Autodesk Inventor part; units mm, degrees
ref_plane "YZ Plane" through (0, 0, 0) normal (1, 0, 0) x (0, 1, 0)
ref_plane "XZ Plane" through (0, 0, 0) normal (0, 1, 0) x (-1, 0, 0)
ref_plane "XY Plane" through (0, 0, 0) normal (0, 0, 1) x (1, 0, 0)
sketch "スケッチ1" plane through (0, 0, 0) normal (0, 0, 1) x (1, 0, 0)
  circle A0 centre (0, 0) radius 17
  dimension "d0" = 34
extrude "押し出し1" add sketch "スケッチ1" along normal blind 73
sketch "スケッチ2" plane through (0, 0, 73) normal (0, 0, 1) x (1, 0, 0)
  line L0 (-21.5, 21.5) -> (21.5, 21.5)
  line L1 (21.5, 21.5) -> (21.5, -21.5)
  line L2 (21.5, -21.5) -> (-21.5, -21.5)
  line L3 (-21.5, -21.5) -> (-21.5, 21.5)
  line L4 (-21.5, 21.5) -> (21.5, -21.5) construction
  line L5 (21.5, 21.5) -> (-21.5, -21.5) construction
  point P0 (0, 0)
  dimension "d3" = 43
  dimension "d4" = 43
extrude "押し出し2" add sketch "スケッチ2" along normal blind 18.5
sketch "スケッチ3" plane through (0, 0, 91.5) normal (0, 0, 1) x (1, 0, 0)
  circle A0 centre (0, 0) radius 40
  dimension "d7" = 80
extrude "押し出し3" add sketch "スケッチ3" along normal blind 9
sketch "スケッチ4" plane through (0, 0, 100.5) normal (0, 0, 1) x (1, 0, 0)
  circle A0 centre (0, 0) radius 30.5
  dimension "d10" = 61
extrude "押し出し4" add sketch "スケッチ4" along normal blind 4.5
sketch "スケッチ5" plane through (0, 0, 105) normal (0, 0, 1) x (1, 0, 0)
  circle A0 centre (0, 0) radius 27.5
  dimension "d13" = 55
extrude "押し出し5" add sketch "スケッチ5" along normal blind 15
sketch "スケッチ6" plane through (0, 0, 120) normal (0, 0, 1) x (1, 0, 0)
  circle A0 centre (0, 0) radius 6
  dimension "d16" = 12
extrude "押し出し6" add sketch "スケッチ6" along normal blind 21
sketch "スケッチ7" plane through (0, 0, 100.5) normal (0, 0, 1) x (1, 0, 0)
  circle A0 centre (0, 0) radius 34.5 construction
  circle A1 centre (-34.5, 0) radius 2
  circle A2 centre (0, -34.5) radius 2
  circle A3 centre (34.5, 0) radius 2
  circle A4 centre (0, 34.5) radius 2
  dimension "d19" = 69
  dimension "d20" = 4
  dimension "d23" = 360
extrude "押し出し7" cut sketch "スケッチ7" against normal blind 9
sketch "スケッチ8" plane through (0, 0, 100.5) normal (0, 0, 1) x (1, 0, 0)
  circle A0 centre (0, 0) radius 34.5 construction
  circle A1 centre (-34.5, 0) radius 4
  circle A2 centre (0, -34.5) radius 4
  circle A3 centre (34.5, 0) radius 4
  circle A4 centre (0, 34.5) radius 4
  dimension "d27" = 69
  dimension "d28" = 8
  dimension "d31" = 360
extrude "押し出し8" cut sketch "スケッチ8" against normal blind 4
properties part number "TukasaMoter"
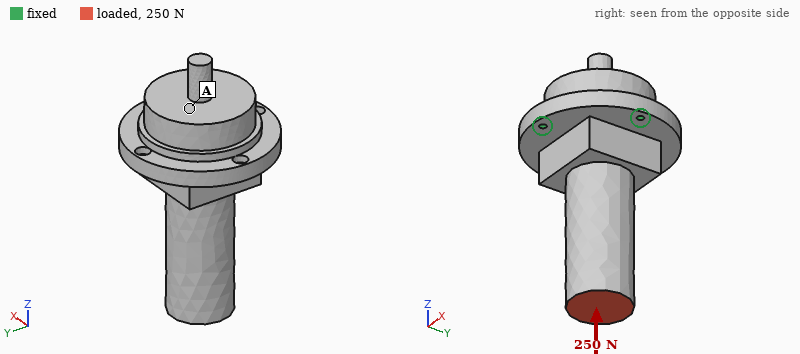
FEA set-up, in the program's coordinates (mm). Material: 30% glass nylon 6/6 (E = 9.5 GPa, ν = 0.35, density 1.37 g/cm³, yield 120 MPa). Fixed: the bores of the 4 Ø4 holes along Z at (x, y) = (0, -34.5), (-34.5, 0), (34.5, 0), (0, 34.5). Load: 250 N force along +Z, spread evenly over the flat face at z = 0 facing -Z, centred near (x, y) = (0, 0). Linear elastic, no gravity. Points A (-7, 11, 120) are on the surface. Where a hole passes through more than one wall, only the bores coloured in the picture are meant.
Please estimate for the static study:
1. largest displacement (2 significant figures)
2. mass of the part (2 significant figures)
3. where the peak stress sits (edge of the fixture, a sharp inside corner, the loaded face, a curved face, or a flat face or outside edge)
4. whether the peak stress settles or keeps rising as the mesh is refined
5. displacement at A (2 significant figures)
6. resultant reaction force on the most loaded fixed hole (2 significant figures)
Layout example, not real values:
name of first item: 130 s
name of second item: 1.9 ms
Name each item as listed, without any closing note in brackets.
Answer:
largest displacement: 4.8 µm
mass of the part: 270 g
where the peak stress sits: edge of the fixture
whether the peak stress settles or keeps rising as the mesh is refined: keeps rising
displacement at A: 2.2 µm
resultant reaction force on the most loaded fixed hole: 66 N
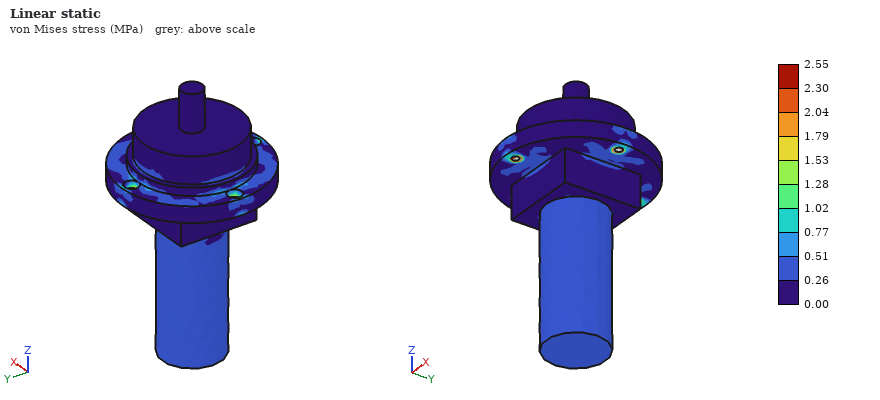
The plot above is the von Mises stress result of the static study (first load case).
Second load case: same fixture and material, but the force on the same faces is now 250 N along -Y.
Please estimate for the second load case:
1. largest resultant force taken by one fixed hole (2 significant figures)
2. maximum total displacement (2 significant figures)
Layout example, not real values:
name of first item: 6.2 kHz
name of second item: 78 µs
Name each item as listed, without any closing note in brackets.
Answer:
largest resultant force taken by one fixed hole: 350 N
maximum total displacement: 0.13 mm
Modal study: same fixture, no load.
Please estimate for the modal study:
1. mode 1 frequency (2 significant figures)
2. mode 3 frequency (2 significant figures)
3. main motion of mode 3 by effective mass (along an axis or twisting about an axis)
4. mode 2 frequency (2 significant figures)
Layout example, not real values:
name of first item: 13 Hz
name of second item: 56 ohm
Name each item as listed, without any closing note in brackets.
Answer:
mode 1 frequency: 1300 Hz
mode 3 frequency: 3200 Hz
main motion of mode 3 by effective mass: along Z
mode 2 frequency: 1300 Hz
